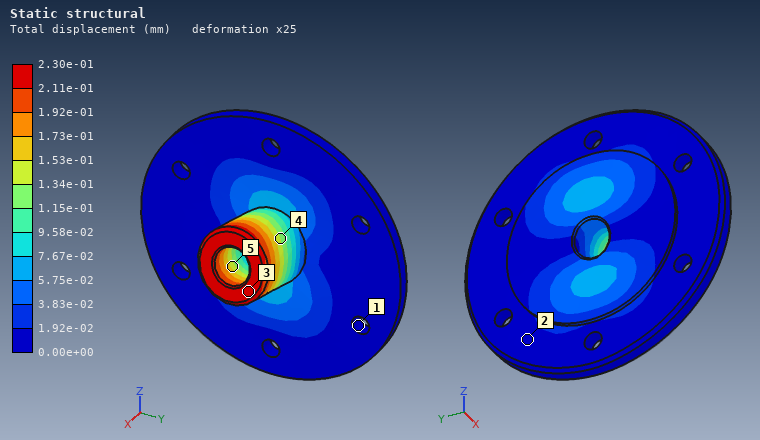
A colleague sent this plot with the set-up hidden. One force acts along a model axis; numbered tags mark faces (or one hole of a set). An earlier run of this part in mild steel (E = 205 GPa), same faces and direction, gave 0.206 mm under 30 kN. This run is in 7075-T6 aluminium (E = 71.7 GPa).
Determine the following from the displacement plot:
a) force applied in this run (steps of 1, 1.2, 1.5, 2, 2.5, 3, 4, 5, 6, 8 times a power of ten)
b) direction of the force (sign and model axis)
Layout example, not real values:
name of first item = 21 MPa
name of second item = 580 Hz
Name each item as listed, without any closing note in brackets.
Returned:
force applied in this run = 12 kN
direction of the force = +Z
